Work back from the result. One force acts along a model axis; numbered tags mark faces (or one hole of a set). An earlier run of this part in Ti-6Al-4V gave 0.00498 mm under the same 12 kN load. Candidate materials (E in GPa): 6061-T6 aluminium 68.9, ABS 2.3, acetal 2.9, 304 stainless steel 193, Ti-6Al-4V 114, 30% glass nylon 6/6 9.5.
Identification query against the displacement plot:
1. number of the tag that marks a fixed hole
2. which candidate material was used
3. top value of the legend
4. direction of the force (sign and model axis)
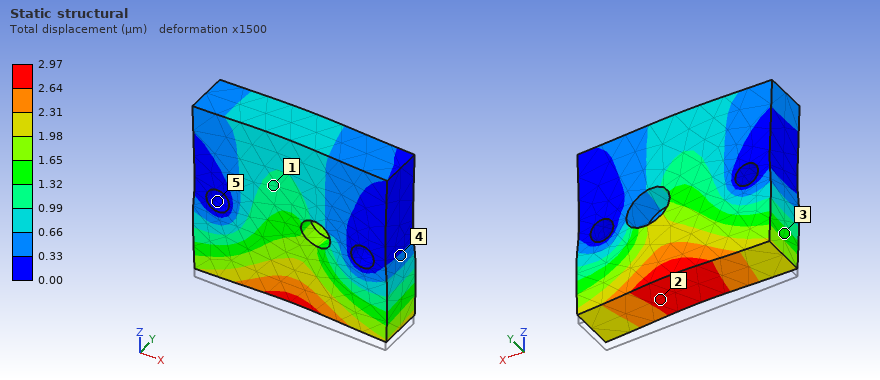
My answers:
5
304 stainless steel
2.97 µm
+Z
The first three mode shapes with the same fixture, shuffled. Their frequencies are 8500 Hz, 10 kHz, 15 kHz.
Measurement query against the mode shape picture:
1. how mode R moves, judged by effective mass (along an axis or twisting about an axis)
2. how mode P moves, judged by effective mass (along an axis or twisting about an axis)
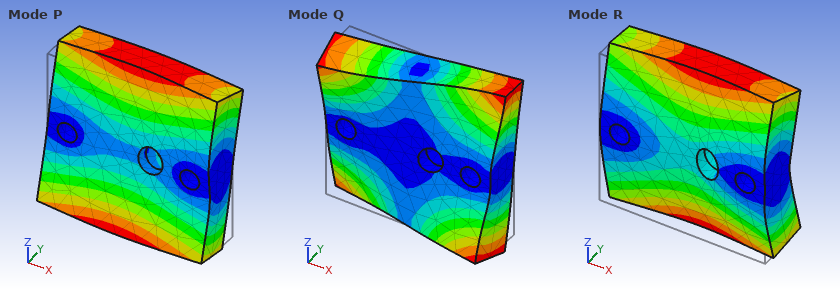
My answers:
along Y
twisting about X
